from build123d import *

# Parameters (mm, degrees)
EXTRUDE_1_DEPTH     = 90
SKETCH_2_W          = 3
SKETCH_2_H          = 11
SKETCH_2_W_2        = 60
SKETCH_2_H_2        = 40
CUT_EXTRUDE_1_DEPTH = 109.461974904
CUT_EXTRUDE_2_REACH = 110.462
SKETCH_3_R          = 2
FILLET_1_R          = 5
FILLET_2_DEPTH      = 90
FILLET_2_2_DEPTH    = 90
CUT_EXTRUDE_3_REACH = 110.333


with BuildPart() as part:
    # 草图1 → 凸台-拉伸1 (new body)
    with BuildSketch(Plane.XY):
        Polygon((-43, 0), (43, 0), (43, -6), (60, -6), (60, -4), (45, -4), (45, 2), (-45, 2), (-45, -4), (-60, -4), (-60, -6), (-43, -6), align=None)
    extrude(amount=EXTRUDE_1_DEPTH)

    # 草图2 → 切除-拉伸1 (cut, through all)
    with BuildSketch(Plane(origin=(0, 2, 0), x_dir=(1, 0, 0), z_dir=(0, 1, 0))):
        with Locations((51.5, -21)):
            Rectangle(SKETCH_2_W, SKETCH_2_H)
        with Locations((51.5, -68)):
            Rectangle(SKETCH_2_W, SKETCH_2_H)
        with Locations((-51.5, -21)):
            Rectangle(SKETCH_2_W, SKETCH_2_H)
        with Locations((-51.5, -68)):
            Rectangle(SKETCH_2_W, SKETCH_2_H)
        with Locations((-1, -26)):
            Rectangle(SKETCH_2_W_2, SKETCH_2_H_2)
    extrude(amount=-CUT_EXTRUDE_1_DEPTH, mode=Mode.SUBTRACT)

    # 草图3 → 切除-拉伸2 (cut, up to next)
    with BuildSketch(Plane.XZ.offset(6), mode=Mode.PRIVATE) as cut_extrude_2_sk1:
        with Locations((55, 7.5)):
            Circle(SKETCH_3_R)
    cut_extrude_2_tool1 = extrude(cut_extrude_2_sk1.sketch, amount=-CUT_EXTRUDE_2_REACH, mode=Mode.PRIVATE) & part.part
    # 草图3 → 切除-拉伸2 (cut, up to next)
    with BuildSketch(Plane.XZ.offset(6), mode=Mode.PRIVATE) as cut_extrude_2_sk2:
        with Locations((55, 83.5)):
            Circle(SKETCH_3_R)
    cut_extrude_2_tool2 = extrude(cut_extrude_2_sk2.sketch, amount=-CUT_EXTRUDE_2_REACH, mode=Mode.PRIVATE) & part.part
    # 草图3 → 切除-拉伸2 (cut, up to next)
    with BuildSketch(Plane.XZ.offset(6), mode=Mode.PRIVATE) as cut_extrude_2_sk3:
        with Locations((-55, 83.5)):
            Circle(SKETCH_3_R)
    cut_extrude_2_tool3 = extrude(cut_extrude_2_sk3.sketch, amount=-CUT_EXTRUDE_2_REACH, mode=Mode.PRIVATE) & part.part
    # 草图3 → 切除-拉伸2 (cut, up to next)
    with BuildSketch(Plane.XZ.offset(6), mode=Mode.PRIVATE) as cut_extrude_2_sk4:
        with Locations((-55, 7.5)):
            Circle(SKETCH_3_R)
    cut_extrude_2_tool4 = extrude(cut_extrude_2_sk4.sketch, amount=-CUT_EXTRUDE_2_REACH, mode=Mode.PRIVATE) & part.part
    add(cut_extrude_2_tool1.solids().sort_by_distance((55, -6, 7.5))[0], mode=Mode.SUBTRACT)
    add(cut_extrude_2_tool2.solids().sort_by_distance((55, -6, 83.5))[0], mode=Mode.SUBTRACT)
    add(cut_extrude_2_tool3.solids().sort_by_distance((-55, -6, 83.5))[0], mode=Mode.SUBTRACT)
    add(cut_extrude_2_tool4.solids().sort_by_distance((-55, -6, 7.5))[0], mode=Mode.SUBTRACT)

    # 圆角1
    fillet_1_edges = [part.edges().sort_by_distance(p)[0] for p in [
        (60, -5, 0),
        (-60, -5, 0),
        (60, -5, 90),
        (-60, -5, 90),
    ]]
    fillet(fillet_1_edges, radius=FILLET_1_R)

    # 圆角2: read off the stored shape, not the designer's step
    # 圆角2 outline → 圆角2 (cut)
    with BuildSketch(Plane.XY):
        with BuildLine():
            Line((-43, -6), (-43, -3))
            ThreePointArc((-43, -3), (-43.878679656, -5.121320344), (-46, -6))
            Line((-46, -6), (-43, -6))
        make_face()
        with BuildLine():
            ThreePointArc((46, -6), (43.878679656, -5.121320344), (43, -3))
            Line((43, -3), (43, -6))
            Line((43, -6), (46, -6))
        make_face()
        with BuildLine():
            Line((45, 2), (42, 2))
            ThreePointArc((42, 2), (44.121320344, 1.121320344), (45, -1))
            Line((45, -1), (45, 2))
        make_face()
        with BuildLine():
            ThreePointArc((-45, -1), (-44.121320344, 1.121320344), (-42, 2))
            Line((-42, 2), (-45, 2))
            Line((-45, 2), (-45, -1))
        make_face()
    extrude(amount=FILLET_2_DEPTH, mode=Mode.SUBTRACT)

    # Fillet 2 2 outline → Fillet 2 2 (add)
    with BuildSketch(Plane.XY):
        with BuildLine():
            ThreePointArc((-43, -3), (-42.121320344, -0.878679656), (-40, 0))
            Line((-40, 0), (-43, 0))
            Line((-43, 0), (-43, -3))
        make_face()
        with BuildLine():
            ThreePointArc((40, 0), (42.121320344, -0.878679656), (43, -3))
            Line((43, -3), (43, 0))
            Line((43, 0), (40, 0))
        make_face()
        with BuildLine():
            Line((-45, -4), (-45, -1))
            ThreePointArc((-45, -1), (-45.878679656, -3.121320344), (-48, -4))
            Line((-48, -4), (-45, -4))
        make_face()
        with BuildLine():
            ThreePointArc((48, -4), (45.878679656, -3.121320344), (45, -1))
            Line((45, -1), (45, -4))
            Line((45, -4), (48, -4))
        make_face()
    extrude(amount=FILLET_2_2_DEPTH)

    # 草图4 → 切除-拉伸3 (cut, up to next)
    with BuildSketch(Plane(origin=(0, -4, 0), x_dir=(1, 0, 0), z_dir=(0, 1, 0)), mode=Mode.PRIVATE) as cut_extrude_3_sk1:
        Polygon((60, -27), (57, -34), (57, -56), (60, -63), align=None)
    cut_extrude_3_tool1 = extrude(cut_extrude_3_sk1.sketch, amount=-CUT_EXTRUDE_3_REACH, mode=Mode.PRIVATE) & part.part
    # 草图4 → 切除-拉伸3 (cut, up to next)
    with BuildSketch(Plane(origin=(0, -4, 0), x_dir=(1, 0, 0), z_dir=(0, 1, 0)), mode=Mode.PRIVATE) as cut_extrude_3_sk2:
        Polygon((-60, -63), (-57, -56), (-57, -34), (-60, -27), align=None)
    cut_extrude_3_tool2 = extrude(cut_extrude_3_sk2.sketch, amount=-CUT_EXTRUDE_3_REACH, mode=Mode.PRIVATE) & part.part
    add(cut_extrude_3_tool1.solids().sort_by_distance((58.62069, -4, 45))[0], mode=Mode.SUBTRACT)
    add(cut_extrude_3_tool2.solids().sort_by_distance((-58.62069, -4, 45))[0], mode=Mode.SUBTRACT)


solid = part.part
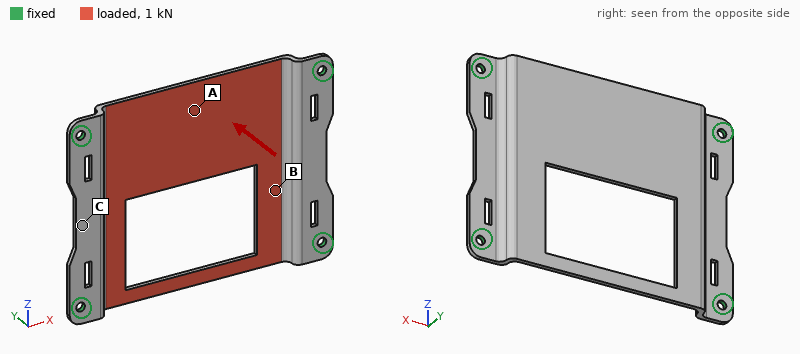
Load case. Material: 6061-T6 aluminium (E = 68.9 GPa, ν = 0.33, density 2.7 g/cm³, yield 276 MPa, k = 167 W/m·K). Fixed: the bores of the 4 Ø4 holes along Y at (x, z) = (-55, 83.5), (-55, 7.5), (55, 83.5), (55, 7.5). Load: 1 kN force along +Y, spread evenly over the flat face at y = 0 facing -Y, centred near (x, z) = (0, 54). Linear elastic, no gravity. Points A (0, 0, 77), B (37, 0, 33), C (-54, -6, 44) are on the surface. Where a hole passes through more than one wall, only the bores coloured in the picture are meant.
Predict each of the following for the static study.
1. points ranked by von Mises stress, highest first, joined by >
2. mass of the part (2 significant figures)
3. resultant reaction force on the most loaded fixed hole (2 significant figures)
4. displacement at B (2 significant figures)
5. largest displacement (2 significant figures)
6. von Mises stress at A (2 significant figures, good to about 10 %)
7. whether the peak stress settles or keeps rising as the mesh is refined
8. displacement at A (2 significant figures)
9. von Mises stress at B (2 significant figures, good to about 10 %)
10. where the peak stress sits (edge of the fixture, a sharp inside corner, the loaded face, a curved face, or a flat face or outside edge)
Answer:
A > B > C
49 g
1.2 kN
0.12 mm
0.74 mm
75 MPa
keeps rising
0.69 mm
41 MPa
edge of the fixture
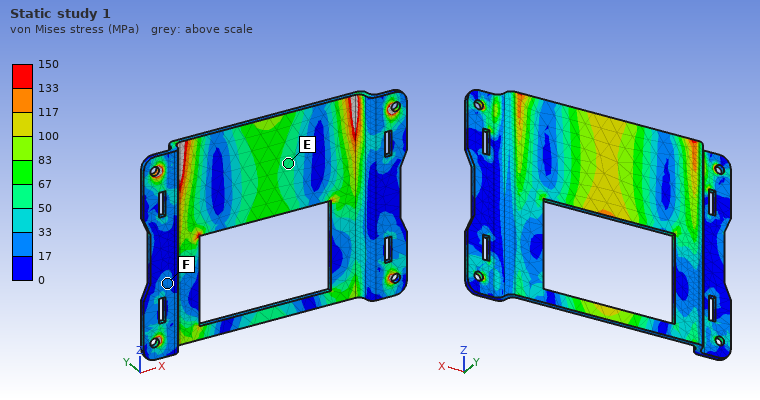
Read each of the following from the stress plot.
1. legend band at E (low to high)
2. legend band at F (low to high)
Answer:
50 to 67 MPa
17 to 33 MPa
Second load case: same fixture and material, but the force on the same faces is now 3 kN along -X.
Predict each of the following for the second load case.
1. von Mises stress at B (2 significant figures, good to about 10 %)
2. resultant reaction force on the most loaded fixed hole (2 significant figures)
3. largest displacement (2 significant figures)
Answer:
28 MPa
1.0 kN
0.40 mm
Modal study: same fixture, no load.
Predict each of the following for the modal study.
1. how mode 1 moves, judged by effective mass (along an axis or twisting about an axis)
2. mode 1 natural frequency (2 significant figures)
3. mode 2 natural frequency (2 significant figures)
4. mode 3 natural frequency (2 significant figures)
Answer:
along Y
1400 Hz
1700 Hz
1800 Hz
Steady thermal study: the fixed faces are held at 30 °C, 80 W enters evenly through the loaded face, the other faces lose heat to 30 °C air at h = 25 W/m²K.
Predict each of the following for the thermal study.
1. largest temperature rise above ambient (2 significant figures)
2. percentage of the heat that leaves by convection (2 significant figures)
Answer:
81 K
18 %
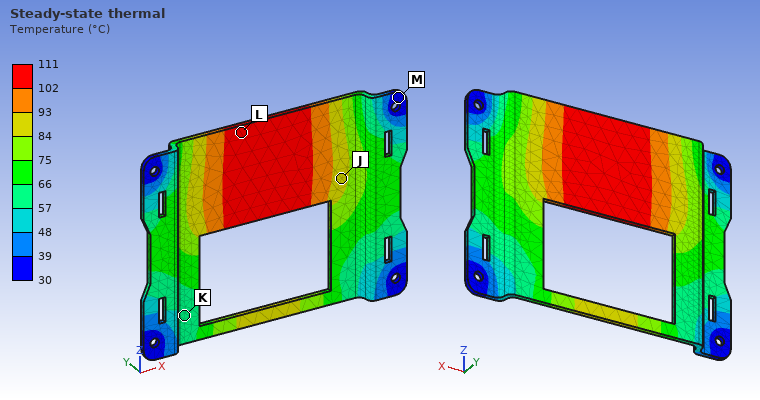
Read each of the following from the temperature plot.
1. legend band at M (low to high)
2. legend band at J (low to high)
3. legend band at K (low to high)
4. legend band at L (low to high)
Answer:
30 to 39 °C
84 to 93 °C
57 to 66 °C
102 to 111 °C
